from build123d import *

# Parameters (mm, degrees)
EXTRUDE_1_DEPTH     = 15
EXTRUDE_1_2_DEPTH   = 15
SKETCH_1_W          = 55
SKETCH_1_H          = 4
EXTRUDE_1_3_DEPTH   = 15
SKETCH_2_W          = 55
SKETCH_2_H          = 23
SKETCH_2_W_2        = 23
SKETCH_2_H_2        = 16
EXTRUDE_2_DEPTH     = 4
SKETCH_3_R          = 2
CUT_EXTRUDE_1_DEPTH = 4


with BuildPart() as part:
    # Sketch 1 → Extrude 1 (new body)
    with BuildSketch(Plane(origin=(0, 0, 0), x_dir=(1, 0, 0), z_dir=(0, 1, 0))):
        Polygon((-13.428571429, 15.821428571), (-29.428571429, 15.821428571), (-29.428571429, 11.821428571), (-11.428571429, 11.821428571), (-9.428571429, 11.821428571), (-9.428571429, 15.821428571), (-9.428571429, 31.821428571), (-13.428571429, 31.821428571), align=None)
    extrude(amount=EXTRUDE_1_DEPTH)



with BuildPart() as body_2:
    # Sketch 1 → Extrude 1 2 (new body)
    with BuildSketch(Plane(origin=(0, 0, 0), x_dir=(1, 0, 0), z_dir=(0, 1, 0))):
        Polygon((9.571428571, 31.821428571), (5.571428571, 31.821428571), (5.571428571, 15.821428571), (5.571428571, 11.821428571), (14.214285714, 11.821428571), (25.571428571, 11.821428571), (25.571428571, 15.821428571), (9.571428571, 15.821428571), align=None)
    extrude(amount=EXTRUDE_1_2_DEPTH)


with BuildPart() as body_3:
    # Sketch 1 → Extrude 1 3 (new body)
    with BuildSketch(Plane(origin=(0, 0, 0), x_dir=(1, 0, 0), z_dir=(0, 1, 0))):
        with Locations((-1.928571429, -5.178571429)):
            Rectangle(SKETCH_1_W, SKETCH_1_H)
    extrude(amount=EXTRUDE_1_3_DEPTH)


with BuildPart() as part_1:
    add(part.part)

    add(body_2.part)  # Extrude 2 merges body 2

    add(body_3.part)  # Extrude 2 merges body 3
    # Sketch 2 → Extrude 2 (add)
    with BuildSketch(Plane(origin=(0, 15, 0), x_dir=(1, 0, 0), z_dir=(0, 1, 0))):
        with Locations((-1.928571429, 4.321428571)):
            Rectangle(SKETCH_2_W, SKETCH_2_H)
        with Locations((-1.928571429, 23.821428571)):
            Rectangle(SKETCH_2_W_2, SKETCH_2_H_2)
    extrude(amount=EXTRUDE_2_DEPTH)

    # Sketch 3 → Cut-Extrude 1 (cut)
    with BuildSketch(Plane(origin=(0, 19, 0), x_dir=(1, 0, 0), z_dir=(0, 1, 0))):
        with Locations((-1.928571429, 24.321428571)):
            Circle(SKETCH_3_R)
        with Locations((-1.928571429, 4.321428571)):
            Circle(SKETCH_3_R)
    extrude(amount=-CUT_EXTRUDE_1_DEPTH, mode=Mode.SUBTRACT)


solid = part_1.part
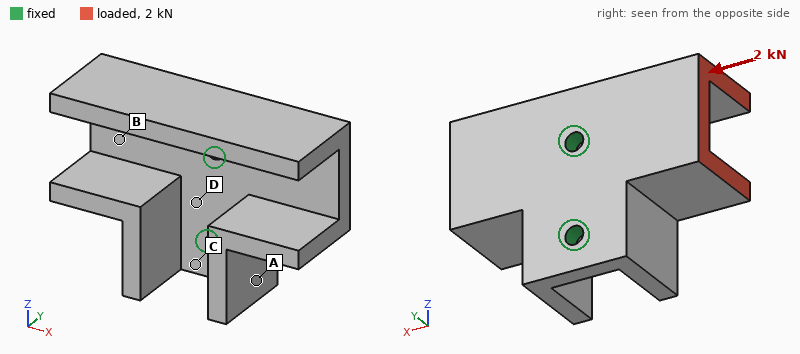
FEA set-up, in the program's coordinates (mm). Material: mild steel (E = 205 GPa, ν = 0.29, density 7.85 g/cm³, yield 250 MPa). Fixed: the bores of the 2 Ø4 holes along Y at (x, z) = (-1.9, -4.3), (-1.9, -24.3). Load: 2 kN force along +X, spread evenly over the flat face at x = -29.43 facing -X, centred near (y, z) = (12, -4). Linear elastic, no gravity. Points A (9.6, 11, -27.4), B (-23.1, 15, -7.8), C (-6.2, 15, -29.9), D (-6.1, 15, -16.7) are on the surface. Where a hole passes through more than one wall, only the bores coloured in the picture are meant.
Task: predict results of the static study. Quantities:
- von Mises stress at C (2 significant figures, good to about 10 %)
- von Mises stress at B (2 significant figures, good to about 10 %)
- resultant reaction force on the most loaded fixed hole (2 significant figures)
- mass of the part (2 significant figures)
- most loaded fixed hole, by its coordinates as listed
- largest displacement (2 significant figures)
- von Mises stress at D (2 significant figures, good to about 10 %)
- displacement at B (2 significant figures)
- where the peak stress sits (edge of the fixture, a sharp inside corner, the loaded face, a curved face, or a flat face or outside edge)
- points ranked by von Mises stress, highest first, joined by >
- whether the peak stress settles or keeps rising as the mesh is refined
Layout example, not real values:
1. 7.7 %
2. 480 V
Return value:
1. 39 MPa
2. 20 MPa
3. 1.9 kN
4. 110 g
5. (-1.9, -4.3)
6. 51 µm
7. 55 MPa
8. 27 µm
9. edge of the fixture
10. D > C > B > A
11. keeps rising
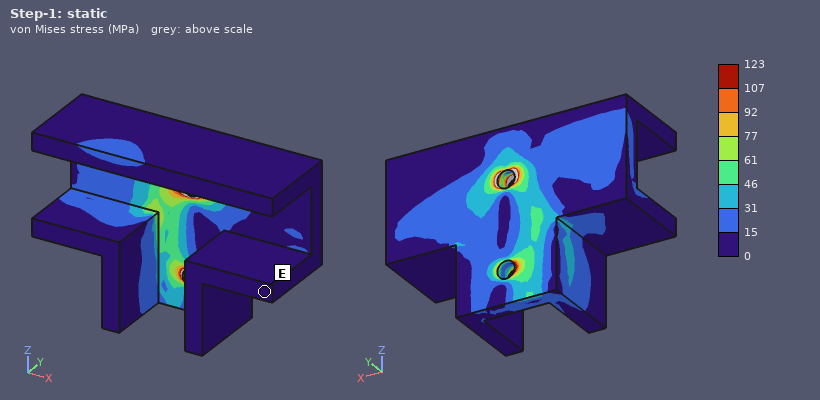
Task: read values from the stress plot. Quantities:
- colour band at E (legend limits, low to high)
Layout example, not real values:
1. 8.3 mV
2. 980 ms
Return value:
1. 0 to 15 MPa
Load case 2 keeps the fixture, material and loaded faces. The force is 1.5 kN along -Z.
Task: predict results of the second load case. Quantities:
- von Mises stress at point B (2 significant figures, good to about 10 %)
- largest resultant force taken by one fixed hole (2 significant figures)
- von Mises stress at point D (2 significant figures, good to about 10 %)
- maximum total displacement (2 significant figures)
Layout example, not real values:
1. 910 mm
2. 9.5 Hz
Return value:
1. 74 MPa
2. 2.0 kN
3. 43 MPa
4. 65 µm
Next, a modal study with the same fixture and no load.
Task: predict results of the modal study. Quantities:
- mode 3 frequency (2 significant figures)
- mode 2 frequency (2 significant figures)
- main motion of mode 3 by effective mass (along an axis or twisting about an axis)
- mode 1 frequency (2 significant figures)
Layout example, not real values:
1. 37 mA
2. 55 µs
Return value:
1. 5800 Hz
2. 4800 Hz
3. along Y
4. 3000 Hz
